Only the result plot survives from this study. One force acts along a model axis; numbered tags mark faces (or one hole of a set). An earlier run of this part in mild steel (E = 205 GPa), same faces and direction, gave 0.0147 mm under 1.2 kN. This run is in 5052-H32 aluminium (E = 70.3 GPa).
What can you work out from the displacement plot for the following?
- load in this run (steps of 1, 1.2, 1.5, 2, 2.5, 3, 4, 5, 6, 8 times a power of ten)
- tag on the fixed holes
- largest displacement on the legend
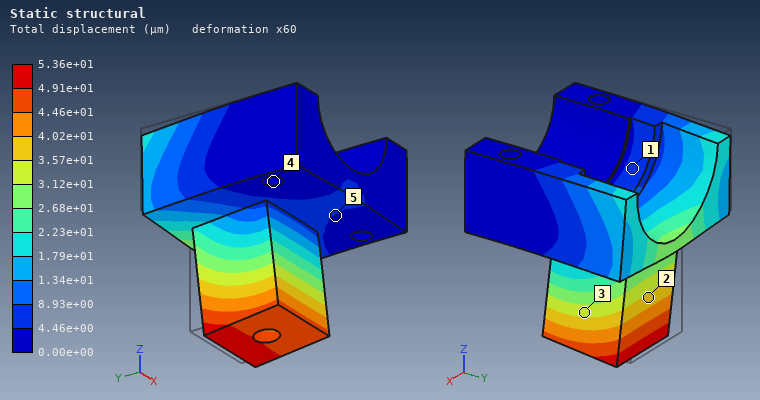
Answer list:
1.5 kN
4
5.36e+01 µm
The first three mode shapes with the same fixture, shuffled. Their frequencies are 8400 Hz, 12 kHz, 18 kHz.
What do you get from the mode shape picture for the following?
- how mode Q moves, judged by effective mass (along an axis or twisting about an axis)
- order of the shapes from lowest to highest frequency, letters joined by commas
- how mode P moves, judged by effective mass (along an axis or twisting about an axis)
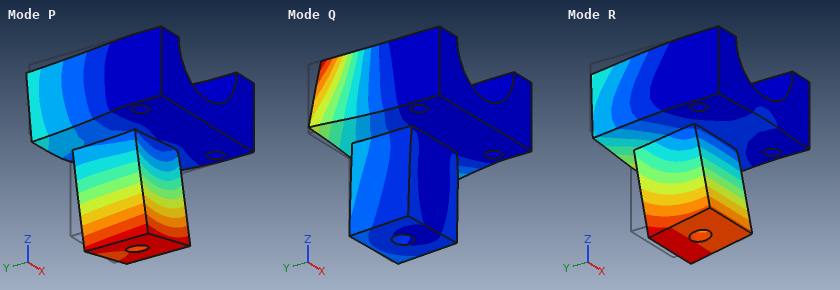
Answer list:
along X
R, P, Q
along X
